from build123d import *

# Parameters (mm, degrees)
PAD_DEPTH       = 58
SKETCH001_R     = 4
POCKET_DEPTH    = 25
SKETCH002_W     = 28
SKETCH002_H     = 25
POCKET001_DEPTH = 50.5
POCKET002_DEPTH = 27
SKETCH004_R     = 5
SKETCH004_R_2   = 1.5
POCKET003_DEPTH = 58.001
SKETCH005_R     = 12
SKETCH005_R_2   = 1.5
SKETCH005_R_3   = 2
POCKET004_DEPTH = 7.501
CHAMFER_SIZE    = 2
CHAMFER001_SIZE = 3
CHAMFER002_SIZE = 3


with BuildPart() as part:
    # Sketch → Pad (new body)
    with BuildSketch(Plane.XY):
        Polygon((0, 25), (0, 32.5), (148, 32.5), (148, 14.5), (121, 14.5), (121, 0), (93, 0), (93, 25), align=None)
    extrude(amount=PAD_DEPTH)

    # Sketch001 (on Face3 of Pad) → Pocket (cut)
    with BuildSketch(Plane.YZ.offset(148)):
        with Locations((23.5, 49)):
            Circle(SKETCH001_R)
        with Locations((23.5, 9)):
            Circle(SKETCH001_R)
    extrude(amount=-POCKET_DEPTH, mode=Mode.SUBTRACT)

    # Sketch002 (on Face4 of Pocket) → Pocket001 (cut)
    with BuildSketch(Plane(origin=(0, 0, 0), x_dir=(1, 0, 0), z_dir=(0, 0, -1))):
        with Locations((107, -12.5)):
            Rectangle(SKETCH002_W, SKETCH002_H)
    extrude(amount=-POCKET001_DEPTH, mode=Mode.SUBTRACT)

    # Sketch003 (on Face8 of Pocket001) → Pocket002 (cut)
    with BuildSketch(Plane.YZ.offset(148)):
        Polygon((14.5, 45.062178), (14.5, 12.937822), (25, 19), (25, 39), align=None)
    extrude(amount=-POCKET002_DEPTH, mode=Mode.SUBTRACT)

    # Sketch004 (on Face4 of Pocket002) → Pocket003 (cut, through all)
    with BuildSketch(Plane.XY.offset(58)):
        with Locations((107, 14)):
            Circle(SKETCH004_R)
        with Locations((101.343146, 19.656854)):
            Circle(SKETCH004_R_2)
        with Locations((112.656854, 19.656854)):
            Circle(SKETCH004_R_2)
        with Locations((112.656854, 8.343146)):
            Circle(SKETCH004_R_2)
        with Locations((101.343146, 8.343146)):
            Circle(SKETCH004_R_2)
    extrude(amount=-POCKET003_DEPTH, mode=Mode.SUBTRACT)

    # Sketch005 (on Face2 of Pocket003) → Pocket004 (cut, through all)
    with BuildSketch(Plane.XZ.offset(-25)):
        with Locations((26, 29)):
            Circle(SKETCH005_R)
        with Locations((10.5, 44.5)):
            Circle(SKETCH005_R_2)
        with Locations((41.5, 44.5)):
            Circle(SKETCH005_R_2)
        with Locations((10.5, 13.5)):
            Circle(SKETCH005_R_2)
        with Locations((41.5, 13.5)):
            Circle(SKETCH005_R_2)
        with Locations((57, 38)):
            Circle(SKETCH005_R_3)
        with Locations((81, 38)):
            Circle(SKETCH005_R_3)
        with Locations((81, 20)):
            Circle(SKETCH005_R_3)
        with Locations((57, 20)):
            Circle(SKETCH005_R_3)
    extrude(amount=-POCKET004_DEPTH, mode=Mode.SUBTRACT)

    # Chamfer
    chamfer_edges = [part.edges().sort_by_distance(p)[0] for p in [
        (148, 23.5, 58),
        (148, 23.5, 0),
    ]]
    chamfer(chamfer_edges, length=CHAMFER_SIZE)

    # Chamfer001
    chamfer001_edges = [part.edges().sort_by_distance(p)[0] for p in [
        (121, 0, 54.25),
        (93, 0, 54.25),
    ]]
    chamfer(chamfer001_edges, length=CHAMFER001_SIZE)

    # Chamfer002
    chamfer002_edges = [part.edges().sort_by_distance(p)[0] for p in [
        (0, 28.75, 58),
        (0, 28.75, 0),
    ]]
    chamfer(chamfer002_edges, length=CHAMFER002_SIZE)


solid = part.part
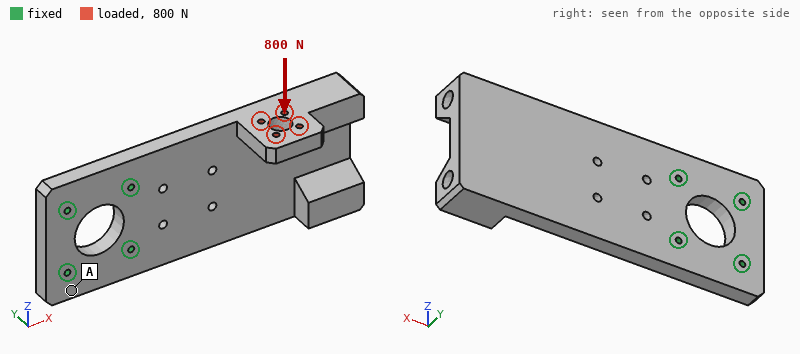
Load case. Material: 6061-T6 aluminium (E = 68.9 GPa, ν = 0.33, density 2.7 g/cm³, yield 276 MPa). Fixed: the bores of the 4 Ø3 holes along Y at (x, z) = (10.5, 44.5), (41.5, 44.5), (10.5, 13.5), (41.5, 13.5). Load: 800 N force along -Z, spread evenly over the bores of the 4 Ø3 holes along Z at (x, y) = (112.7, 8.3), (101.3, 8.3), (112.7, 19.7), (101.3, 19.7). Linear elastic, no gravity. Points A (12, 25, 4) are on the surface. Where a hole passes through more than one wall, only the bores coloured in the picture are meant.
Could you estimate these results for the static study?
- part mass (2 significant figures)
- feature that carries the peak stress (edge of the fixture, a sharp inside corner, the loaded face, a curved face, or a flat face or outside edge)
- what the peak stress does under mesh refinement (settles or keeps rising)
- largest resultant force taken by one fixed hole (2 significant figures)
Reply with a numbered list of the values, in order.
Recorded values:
1. 190 g
2. edge of the fixture
3. keeps rising
4. 1.3 kN
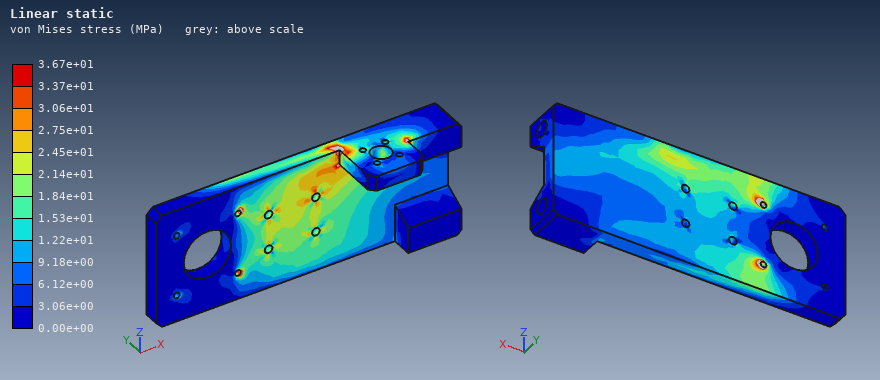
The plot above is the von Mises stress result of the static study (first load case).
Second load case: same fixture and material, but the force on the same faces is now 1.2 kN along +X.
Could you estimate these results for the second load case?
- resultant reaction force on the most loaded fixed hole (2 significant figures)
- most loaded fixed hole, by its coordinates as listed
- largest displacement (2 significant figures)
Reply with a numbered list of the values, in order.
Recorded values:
1. 1.2 kN
2. (41.5, 44.5)
3. 0.71 mm
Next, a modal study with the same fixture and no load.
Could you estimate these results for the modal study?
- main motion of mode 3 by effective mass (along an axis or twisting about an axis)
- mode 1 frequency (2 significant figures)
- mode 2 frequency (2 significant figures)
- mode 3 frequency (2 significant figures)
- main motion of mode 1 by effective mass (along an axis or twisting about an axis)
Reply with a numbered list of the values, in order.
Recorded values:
1. along Z
2. 410 Hz
3. 1500 Hz
4. 2500 Hz
5. along Y
